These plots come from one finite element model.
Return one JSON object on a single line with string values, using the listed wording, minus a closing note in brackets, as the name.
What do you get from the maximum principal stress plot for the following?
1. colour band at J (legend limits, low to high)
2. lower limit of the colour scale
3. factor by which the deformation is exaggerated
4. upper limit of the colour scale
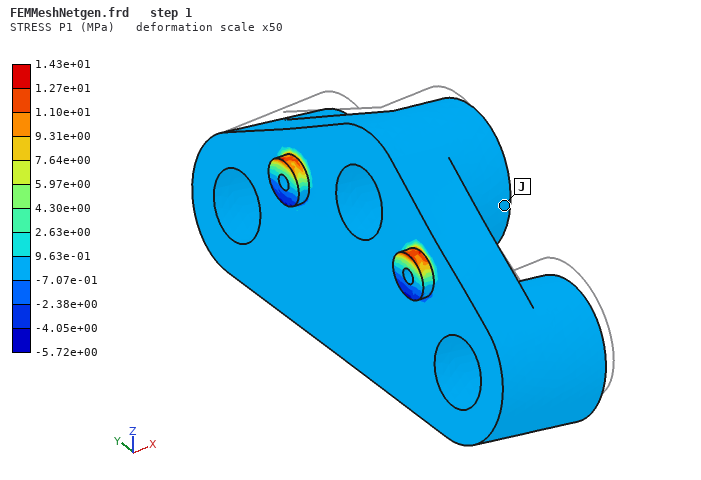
{"colour band at J": "-7.07e-01 to 9.63e-01 MPa", "lower limit of the colour scale": "-5.72e+00 MPa", "factor by which the deformation is exaggerated": "50", "upper limit of the colour scale": "1.43e+01 MPa"}
